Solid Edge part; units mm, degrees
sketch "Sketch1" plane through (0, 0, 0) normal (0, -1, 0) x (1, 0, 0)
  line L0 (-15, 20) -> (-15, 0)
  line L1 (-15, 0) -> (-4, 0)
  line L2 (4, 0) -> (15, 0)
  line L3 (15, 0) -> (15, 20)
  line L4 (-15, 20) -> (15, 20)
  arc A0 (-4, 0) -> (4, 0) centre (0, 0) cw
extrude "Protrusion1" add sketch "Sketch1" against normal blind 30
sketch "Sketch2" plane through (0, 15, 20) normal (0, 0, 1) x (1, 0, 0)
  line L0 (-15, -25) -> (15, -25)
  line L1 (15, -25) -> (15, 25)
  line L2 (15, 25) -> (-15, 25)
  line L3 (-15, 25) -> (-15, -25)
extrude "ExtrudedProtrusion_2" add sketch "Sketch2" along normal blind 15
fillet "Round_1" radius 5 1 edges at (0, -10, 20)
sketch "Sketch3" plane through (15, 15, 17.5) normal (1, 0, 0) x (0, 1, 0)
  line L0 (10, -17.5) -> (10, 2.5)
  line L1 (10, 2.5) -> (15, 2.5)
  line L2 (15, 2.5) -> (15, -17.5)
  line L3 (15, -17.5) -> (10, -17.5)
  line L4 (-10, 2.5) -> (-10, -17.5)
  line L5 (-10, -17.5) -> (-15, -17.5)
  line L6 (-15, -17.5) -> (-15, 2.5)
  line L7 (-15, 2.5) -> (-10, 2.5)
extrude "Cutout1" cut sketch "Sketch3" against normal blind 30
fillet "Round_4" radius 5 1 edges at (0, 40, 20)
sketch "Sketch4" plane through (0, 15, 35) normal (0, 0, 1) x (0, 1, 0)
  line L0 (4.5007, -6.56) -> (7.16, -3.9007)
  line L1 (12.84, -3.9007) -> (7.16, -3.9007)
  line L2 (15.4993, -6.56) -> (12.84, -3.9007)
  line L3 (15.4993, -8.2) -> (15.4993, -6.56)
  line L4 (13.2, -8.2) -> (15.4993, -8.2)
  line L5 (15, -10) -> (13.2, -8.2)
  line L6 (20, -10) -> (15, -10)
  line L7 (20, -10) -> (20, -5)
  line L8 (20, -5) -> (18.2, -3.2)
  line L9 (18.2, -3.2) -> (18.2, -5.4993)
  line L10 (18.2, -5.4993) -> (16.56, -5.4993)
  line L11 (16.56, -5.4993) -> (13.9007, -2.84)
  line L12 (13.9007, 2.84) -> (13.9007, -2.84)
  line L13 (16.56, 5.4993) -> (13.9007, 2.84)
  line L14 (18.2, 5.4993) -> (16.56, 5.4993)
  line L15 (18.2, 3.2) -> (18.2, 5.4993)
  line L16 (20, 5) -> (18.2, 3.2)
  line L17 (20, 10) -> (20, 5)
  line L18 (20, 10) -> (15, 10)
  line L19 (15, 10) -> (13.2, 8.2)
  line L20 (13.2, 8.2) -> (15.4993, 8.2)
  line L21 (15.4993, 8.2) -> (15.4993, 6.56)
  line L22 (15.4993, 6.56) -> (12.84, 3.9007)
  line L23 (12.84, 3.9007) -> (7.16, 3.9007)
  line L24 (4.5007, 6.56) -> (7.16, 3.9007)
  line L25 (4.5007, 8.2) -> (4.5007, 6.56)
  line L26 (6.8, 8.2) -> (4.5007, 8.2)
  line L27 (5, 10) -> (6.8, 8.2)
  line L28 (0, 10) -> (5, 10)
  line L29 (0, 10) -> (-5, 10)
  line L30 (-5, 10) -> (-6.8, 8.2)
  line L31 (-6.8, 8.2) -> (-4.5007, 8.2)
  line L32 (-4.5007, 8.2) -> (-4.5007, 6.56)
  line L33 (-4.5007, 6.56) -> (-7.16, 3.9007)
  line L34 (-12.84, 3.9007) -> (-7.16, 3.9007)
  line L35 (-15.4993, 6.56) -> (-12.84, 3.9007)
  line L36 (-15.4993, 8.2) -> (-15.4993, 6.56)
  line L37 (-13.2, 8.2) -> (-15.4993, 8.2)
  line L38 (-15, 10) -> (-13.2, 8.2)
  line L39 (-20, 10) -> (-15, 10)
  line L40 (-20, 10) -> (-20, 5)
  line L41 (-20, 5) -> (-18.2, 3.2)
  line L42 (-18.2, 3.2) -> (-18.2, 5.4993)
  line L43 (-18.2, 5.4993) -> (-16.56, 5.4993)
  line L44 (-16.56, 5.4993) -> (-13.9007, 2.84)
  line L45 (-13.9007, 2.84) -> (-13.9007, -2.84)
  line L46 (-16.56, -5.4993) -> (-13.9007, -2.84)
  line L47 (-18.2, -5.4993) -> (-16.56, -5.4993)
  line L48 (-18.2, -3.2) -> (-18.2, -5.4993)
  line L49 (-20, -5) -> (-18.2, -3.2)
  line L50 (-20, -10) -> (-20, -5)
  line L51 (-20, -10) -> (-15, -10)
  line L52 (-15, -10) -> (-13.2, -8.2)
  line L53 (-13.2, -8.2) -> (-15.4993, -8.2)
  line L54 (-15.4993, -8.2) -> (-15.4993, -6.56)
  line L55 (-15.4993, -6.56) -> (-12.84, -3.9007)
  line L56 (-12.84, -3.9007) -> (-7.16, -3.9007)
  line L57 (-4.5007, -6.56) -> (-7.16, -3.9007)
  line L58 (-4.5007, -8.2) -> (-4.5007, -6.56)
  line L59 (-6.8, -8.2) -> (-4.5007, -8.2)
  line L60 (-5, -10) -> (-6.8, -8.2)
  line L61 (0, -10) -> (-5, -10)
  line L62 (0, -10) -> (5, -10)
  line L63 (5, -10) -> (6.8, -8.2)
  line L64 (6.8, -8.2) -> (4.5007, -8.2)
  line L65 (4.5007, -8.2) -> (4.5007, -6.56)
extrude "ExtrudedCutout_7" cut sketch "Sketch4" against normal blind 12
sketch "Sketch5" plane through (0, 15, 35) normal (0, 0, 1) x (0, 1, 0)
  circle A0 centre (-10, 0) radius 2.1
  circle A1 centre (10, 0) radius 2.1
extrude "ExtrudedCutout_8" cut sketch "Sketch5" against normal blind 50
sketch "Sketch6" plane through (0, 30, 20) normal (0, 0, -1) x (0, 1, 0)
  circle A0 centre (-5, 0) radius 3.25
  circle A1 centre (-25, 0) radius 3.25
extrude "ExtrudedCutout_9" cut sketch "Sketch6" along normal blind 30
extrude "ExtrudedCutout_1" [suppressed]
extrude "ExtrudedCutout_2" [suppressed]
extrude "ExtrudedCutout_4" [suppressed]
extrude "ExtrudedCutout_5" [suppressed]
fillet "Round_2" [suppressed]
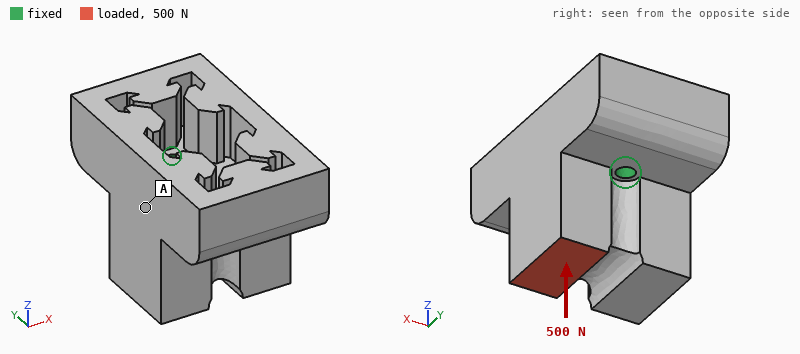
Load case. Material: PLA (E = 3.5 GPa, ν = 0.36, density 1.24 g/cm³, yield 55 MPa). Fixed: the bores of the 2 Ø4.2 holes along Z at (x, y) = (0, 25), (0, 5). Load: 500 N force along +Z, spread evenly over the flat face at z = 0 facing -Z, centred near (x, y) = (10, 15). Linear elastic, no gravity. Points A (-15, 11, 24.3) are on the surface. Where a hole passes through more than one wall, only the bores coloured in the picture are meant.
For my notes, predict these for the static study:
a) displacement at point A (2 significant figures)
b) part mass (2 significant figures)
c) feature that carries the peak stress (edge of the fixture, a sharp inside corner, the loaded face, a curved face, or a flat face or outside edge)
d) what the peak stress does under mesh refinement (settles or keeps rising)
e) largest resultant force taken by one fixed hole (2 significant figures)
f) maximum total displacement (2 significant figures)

0.24 mm
34 g
edge of the fixture
keeps rising
260 N
0.47 mm
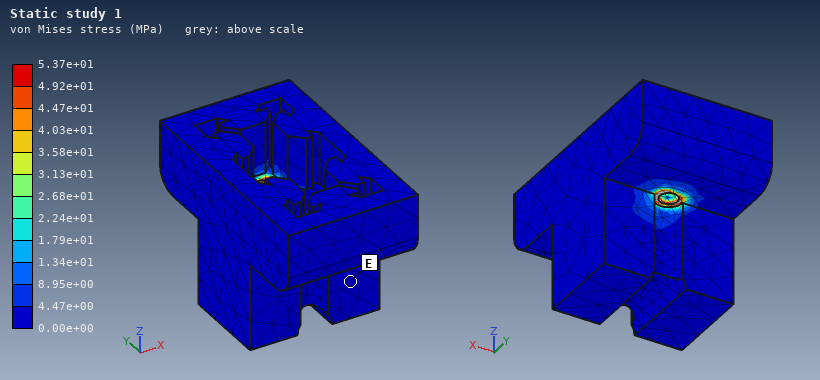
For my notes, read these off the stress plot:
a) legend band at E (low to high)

0.00e+00 to 4.47e+00 MPa
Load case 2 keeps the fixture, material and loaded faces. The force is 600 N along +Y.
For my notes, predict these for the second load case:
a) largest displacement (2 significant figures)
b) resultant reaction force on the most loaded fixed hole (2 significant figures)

0.22 mm
760 N
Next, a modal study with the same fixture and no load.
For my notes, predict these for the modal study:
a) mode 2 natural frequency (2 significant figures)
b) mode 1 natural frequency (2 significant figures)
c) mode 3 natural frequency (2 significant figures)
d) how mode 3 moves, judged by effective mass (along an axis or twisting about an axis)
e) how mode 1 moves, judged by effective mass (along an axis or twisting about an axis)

2800 Hz
1100 Hz
4000 Hz
twisting about Z
twisting about Y
